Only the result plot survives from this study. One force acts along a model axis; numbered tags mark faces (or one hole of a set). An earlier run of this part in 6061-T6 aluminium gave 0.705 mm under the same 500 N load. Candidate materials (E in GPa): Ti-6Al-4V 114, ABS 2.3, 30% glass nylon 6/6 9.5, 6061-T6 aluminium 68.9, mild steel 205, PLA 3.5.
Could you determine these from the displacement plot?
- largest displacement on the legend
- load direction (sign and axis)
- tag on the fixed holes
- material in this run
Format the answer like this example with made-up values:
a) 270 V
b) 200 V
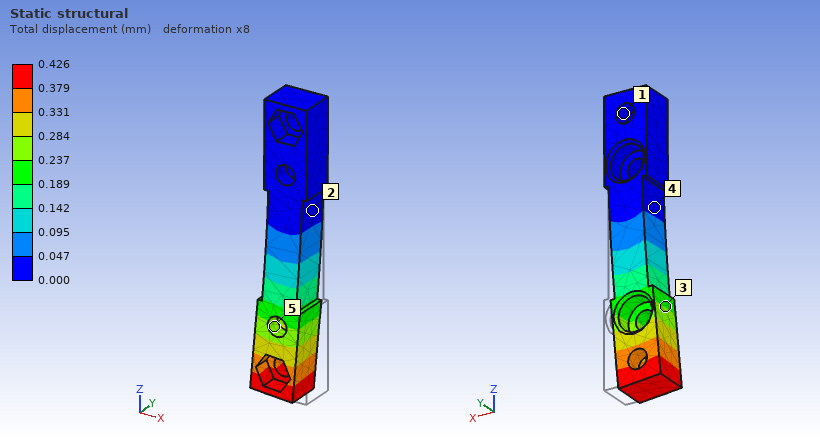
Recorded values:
a) 0.426 mm
b) -X
c) 1
d) Ti-6Al-4V
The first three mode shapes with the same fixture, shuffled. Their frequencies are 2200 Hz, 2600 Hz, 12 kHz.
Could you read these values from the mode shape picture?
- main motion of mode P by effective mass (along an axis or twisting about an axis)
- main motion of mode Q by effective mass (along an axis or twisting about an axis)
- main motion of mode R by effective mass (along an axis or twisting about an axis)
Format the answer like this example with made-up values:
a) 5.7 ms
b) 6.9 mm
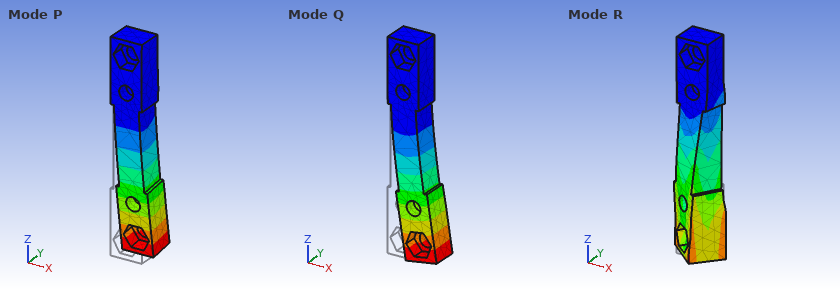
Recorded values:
a) along Y
b) along X
c) twisting about Z
